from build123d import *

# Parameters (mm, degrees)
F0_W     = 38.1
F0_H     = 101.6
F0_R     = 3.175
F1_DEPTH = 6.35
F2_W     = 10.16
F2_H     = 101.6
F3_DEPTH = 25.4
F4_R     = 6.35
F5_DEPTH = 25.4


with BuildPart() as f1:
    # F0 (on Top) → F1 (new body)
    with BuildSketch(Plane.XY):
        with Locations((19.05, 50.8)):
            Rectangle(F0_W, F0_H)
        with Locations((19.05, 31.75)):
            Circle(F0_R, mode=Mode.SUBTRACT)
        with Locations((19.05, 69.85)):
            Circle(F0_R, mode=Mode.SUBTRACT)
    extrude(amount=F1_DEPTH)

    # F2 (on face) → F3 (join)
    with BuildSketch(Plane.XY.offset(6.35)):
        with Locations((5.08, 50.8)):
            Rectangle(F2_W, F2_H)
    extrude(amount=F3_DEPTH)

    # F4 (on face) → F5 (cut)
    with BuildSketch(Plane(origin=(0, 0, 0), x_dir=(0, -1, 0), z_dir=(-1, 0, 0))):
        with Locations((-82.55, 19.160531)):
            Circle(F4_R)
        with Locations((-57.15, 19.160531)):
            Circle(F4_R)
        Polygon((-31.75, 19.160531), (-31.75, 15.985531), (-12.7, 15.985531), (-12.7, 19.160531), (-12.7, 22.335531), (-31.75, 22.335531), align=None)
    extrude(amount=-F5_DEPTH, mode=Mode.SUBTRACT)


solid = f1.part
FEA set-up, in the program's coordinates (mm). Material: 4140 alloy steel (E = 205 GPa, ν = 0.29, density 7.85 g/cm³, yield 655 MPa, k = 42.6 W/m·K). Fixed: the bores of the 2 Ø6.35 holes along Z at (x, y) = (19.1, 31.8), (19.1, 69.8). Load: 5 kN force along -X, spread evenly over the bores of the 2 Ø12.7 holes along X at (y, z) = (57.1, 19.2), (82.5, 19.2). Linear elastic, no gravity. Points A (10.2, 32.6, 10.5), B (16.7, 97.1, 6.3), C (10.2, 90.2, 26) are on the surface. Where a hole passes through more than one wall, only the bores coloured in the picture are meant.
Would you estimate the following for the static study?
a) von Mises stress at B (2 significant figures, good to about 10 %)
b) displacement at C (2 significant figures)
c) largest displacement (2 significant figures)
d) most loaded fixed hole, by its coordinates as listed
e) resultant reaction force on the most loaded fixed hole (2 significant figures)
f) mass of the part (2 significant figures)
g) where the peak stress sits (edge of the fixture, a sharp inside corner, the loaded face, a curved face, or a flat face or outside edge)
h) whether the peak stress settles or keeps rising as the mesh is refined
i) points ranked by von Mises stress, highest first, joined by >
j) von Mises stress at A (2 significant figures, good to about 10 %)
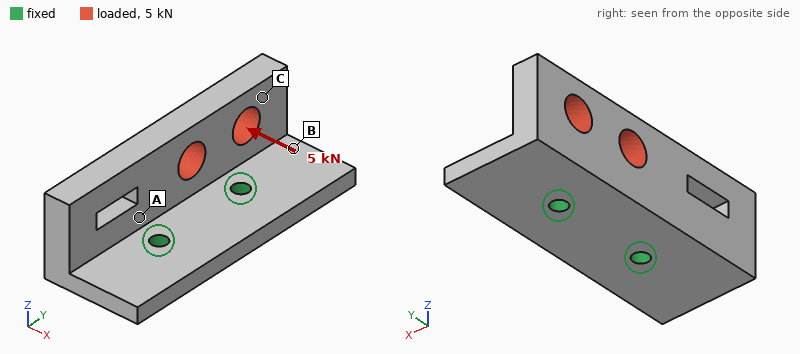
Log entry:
77 MPa
0.091 mm
0.13 mm
(19.1, 69.8)
4.8 kN
370 g
edge of the fixture
keeps rising
B > A > C
48 MPa
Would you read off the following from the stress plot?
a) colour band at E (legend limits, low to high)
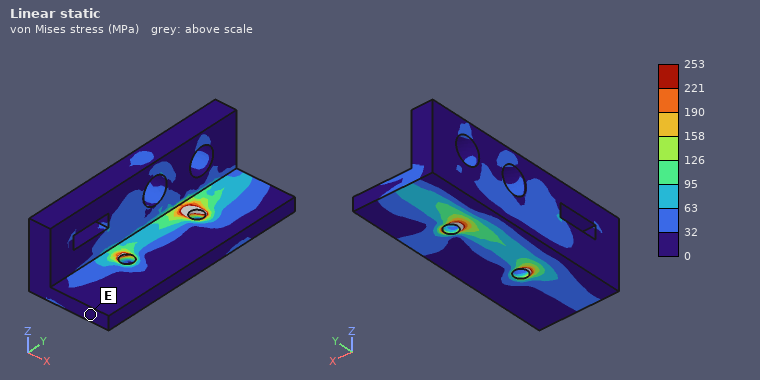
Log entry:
0 to 32 MPa
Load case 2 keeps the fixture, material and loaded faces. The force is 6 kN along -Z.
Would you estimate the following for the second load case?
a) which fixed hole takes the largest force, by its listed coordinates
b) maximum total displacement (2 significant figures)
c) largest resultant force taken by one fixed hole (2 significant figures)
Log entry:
(19.1, 69.8)
92 µm
5.5 kN
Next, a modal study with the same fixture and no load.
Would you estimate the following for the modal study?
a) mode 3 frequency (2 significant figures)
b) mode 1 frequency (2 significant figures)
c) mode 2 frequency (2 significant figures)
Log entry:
5900 Hz
3000 Hz
4000 Hz
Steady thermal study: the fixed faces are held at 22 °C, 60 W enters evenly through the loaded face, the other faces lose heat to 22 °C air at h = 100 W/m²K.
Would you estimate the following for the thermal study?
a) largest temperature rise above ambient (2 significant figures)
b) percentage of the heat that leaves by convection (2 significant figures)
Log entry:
65 K
51 %
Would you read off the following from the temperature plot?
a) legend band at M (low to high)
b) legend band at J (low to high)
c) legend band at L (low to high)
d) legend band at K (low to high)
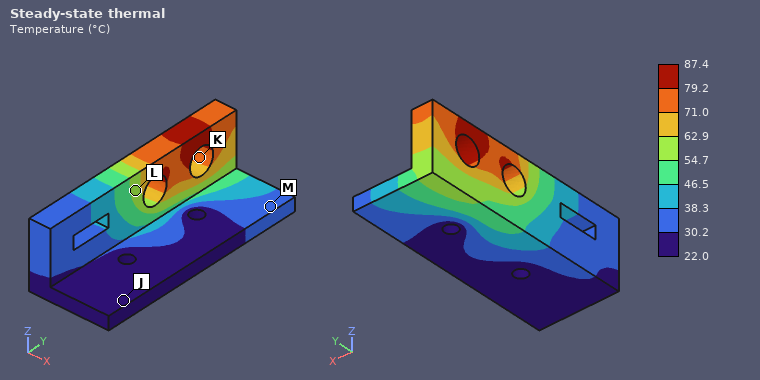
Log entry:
30.2 to 38.3 °C
22.0 to 30.2 °C
54.7 to 62.9 °C
71.0 to 79.2 °C
